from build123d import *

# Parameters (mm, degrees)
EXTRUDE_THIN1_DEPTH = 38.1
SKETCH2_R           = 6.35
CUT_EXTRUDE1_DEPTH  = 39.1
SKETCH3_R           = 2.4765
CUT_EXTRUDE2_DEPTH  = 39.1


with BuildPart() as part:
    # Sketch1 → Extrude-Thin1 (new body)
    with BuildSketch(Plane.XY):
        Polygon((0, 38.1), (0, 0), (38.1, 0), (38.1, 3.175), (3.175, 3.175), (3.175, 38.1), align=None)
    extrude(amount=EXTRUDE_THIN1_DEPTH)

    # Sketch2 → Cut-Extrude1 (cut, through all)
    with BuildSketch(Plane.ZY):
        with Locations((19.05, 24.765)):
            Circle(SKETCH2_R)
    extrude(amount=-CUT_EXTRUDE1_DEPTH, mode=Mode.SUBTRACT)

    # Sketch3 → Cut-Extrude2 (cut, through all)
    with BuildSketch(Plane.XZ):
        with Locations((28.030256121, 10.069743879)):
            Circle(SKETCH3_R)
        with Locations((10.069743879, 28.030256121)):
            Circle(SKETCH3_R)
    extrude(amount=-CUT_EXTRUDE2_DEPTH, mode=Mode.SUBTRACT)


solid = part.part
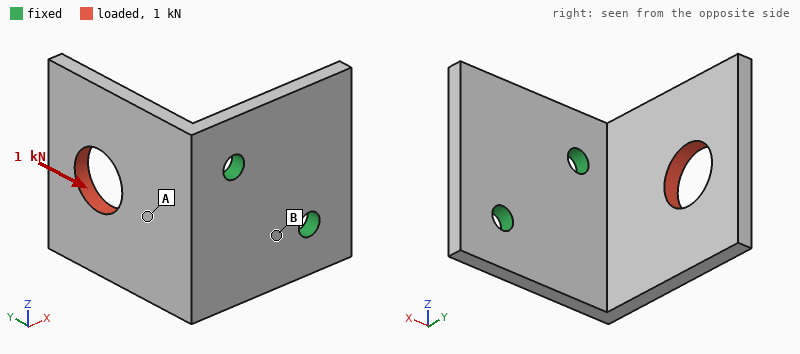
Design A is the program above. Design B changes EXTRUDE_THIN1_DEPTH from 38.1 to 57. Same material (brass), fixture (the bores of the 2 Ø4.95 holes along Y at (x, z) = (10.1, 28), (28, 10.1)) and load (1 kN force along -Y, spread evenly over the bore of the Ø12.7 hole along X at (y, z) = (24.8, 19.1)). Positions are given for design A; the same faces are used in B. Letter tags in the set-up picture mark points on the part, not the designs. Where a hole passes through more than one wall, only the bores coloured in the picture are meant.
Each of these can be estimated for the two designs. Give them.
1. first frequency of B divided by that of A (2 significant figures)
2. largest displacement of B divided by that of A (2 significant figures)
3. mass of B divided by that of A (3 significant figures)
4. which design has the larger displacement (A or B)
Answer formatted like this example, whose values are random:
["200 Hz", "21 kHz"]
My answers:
["0.96", "0.82", "1.53", "A"]
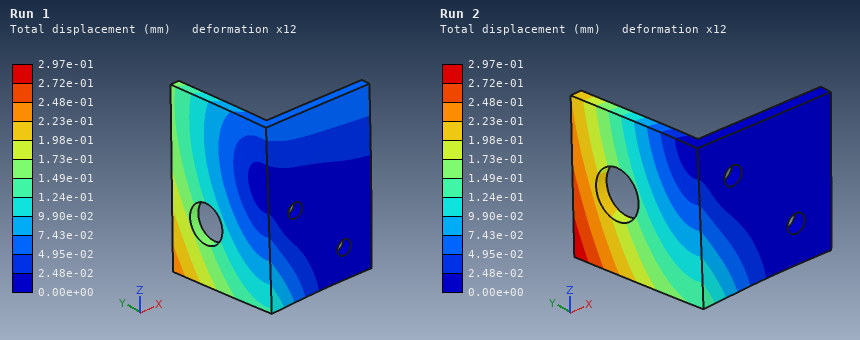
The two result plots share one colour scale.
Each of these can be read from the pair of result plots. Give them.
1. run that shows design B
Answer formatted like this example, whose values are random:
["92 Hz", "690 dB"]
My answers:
["Run 1"]
